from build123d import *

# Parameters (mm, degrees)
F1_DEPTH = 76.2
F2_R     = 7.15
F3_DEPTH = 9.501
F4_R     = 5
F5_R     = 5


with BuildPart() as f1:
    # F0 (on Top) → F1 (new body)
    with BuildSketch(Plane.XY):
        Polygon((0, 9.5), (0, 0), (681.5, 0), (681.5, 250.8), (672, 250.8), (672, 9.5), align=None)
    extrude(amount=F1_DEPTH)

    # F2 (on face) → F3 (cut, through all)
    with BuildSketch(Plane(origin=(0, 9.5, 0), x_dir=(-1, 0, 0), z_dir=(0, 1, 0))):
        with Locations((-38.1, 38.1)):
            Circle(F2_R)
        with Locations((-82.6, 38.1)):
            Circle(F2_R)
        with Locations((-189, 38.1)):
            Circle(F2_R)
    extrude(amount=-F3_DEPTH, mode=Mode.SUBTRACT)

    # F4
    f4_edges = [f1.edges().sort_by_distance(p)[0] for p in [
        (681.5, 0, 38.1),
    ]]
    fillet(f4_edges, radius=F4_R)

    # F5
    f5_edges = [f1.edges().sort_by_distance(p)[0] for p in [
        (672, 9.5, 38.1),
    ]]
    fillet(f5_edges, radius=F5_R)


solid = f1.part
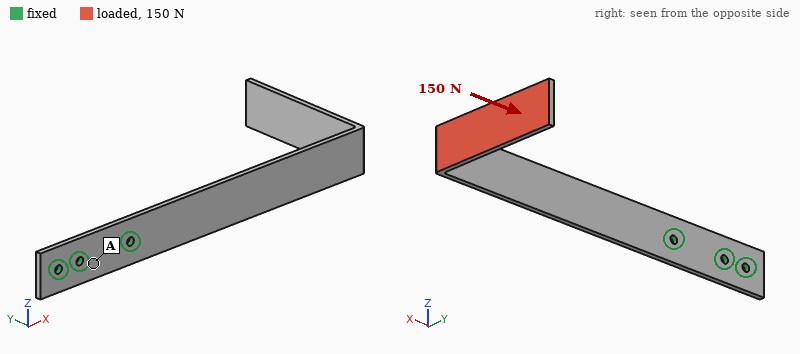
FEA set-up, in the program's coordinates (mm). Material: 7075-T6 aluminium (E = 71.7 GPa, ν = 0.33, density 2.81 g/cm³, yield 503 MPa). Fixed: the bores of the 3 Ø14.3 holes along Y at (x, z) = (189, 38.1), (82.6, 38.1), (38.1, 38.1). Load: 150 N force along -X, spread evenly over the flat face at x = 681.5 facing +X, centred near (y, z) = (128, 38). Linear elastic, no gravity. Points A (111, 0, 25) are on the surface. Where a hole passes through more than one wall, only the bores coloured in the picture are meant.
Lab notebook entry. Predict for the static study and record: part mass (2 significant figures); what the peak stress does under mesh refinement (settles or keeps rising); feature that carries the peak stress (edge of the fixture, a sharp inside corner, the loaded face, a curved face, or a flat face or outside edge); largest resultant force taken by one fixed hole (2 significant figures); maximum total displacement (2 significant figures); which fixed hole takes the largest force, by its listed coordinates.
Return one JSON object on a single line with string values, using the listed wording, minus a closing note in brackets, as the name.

{"part mass": "1.9 kg", "what the peak stress does under mesh refinement": "keeps rising", "feature that carries the peak stress": "edge of the fixture", "largest resultant force taken by one fixed hole": "130 N", "maximum total displacement": "8.4 mm", "which fixed hole takes the largest force, by its listed coordinates": "(189, 38.1)"}
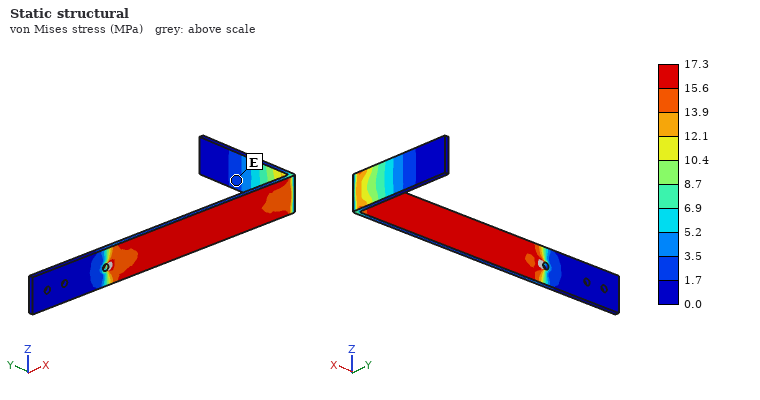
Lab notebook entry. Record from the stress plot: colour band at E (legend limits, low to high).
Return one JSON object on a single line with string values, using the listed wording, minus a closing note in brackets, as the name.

{"colour band at E": "1.7 to 3.5 MPa"}
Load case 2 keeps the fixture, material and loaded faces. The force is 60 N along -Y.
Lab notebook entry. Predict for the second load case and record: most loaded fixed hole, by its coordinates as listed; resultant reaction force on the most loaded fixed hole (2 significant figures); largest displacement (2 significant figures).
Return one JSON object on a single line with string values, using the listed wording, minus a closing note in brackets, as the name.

{"most loaded fixed hole, by its coordinates as listed": "(189, 38.1)", "resultant reaction force on the most loaded fixed hole": "93 N", "largest displacement": "7.6 mm"}
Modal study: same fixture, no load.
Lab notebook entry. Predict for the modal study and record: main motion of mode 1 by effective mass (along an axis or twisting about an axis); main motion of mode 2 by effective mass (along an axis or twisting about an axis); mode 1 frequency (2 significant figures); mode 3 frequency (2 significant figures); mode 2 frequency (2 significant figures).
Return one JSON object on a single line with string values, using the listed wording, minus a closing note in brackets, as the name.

{"main motion of mode 1 by effective mass": "along Y", "main motion of mode 2 by effective mass": "along Z", "mode 1 frequency": "18 Hz", "mode 3 frequency": "73 Hz", "mode 2 frequency": "51 Hz"}
